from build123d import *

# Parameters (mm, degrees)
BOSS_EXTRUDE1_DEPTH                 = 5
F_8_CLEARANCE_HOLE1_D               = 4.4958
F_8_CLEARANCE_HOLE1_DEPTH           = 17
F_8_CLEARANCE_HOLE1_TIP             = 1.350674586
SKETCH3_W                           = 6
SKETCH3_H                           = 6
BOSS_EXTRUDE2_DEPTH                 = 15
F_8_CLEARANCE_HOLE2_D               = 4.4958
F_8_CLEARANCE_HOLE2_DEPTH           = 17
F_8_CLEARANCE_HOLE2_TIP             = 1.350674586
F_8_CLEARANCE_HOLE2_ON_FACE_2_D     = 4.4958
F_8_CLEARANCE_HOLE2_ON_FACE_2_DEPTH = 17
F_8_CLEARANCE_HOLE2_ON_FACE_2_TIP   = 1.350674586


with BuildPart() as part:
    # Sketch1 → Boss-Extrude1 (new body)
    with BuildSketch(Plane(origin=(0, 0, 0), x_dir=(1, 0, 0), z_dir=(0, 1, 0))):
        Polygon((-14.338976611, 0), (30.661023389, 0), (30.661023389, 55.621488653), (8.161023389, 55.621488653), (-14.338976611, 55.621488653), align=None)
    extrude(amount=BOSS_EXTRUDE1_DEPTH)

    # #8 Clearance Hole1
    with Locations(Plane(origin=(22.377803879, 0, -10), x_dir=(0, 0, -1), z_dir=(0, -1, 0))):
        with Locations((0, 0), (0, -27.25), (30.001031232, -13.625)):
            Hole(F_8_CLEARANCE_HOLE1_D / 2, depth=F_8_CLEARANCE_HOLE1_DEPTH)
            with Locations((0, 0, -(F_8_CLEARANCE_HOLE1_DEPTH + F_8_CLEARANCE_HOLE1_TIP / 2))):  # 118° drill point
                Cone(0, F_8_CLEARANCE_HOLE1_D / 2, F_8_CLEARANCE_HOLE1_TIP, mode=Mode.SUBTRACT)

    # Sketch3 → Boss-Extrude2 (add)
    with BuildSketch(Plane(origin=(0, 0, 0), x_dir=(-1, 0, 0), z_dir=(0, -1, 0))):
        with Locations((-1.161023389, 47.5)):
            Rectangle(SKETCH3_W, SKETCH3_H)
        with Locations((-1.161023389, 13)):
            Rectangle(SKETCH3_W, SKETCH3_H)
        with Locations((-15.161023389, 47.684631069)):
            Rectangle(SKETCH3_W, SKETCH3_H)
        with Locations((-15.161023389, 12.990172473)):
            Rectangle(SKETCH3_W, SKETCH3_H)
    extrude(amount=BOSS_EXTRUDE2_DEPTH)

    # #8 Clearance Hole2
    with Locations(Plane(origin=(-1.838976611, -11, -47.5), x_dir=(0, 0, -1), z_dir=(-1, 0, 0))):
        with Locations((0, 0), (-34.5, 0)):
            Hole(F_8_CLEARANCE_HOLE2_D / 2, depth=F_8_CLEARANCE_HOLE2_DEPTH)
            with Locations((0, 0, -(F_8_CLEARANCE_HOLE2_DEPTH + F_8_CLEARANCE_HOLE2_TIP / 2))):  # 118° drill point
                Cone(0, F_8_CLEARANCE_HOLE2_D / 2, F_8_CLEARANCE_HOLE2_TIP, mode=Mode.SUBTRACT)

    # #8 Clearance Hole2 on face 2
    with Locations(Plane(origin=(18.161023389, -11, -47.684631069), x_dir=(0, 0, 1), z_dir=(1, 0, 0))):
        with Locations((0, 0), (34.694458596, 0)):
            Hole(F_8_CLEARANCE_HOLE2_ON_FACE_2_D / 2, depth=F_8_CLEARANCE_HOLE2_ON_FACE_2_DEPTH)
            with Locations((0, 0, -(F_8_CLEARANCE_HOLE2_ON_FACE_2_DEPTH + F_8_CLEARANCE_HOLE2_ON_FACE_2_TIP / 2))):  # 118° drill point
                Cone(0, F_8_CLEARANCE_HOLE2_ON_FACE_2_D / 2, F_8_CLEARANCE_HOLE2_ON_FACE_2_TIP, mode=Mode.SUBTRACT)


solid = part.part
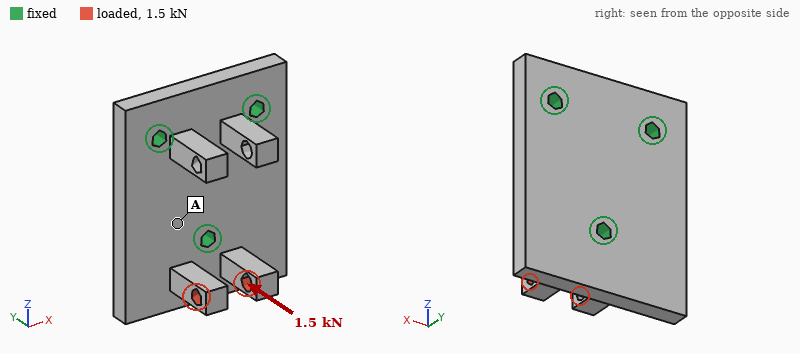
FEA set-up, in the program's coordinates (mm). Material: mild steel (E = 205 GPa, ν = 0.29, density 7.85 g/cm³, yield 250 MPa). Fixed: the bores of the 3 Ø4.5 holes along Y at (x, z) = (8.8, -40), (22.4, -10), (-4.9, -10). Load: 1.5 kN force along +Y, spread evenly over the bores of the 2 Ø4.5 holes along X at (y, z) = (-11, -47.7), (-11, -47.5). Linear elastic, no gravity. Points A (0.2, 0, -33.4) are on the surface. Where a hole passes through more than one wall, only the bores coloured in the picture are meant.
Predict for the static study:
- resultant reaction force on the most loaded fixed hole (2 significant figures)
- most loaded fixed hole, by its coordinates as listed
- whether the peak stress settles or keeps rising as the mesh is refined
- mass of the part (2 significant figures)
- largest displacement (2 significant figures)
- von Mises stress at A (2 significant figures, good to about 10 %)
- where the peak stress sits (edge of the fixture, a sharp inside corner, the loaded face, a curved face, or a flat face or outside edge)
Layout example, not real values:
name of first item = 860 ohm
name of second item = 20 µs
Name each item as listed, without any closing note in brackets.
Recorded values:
resultant reaction force on the most loaded fixed hole = 1.6 kN
most loaded fixed hole, by its coordinates as listed = (8.8, -40)
whether the peak stress settles or keeps rising as the mesh is refined = keeps rising
mass of the part = 110 g
largest displacement = 21 µm
von Mises stress at A = 18 MPa
where the peak stress sits = edge of the fixture
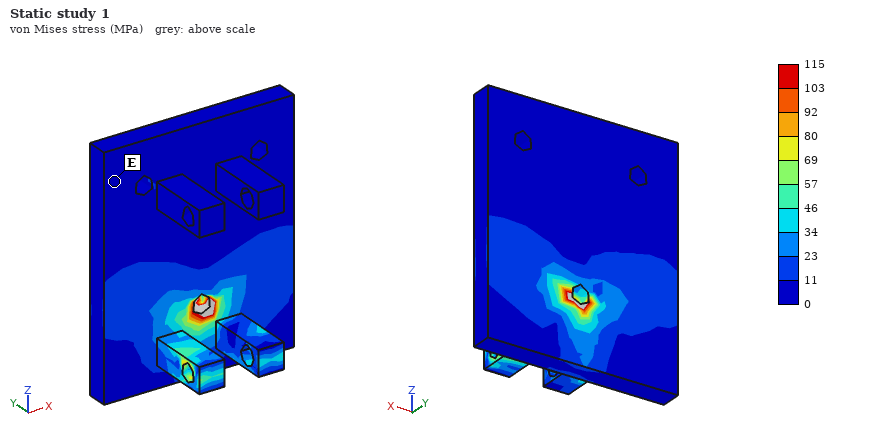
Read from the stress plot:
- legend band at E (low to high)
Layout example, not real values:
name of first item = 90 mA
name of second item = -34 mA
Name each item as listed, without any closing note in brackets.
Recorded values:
legend band at E = 0 to 11 MPa
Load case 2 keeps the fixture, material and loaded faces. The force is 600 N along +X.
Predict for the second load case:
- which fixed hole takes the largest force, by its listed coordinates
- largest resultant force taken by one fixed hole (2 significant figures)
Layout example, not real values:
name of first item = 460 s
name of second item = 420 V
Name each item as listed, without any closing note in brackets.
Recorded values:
which fixed hole takes the largest force, by its listed coordinates = (8.8, -40)
largest resultant force taken by one fixed hole = 640 N
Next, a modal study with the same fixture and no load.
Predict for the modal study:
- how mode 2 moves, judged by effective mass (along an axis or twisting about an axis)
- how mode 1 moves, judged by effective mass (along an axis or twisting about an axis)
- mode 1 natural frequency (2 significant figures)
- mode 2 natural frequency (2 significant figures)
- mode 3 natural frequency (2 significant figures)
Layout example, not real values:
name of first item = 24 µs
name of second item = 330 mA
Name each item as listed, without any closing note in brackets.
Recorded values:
how mode 2 moves, judged by effective mass = along Y
how mode 1 moves, judged by effective mass = twisting about Z
mode 1 natural frequency = 7100 Hz
mode 2 natural frequency = 8400 Hz
mode 3 natural frequency = 12 kHz
